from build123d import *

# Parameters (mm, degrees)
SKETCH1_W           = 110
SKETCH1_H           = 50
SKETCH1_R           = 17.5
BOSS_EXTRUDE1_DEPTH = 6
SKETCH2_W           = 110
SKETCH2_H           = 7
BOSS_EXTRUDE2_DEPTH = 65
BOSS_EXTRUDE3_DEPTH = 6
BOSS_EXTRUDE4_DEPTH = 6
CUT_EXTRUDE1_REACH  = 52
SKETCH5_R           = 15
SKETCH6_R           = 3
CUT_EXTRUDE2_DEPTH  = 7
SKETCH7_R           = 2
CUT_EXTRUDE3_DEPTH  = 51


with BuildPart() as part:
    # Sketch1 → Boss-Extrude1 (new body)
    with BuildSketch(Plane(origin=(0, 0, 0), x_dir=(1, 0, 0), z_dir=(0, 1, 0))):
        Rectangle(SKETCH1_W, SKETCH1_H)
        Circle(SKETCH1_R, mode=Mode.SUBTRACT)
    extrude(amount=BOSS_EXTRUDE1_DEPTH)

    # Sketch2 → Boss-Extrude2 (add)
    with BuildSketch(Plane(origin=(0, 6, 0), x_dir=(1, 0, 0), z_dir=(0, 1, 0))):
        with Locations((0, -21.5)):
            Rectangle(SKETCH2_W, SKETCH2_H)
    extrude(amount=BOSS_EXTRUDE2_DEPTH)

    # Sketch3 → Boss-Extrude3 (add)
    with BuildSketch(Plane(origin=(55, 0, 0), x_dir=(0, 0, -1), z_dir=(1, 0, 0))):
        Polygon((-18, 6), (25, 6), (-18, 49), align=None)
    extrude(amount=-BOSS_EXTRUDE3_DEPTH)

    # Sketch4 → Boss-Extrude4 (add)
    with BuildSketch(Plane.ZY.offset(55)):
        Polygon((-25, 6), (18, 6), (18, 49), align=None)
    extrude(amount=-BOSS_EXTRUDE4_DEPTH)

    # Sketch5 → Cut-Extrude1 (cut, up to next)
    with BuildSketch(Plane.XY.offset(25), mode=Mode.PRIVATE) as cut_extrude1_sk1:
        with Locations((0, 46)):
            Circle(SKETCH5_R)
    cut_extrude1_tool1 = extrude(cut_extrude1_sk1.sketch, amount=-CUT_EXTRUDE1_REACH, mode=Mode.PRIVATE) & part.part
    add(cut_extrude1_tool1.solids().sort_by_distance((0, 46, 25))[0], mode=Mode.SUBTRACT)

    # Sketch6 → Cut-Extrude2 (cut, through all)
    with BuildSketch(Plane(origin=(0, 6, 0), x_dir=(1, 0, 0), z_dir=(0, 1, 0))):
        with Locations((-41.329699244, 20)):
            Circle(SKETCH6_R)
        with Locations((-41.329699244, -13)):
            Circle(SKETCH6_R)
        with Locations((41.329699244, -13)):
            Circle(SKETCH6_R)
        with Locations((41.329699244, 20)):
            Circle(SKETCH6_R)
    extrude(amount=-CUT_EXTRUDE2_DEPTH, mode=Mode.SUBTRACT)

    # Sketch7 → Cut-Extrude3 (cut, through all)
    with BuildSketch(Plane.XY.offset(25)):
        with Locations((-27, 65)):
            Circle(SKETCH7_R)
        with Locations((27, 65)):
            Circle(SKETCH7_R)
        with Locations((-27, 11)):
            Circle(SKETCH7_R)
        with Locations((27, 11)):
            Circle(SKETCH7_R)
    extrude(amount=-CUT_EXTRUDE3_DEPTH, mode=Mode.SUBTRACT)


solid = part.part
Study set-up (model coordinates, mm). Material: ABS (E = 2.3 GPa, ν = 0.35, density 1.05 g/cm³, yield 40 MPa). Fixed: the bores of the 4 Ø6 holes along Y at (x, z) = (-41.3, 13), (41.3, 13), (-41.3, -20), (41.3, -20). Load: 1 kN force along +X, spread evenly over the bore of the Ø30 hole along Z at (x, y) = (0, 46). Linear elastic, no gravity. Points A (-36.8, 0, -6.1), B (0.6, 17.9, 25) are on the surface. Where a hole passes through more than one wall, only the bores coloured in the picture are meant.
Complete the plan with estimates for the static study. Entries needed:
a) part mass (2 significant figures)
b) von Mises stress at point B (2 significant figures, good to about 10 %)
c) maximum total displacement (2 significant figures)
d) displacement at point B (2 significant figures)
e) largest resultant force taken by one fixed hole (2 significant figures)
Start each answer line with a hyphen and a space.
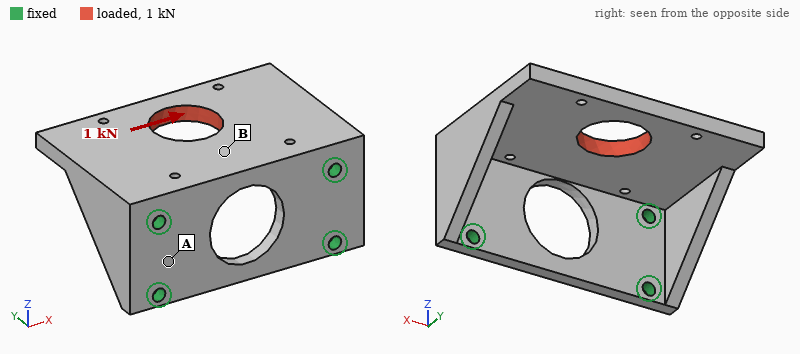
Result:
- 87 g
- 4.1 MPa
- 0.40 mm
- 0.083 mm
- 740 N
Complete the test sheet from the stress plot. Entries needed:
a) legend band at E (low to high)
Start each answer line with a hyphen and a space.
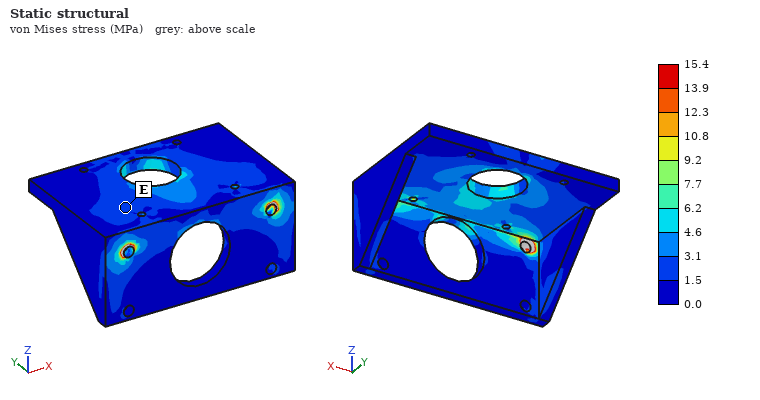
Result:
- 1.5 to 3.1 MPa
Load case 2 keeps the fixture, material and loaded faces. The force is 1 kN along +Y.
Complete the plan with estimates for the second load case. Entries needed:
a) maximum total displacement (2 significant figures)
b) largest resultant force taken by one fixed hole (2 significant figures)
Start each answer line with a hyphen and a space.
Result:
- 0.35 mm
- 590 N
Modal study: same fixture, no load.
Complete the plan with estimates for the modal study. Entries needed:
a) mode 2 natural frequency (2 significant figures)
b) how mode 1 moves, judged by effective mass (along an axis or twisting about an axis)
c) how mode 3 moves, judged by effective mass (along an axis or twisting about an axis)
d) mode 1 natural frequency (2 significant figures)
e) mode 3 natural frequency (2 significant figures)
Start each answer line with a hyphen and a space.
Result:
- 1000 Hz
- along Z
- along X
- 550 Hz
- 1700 Hz
